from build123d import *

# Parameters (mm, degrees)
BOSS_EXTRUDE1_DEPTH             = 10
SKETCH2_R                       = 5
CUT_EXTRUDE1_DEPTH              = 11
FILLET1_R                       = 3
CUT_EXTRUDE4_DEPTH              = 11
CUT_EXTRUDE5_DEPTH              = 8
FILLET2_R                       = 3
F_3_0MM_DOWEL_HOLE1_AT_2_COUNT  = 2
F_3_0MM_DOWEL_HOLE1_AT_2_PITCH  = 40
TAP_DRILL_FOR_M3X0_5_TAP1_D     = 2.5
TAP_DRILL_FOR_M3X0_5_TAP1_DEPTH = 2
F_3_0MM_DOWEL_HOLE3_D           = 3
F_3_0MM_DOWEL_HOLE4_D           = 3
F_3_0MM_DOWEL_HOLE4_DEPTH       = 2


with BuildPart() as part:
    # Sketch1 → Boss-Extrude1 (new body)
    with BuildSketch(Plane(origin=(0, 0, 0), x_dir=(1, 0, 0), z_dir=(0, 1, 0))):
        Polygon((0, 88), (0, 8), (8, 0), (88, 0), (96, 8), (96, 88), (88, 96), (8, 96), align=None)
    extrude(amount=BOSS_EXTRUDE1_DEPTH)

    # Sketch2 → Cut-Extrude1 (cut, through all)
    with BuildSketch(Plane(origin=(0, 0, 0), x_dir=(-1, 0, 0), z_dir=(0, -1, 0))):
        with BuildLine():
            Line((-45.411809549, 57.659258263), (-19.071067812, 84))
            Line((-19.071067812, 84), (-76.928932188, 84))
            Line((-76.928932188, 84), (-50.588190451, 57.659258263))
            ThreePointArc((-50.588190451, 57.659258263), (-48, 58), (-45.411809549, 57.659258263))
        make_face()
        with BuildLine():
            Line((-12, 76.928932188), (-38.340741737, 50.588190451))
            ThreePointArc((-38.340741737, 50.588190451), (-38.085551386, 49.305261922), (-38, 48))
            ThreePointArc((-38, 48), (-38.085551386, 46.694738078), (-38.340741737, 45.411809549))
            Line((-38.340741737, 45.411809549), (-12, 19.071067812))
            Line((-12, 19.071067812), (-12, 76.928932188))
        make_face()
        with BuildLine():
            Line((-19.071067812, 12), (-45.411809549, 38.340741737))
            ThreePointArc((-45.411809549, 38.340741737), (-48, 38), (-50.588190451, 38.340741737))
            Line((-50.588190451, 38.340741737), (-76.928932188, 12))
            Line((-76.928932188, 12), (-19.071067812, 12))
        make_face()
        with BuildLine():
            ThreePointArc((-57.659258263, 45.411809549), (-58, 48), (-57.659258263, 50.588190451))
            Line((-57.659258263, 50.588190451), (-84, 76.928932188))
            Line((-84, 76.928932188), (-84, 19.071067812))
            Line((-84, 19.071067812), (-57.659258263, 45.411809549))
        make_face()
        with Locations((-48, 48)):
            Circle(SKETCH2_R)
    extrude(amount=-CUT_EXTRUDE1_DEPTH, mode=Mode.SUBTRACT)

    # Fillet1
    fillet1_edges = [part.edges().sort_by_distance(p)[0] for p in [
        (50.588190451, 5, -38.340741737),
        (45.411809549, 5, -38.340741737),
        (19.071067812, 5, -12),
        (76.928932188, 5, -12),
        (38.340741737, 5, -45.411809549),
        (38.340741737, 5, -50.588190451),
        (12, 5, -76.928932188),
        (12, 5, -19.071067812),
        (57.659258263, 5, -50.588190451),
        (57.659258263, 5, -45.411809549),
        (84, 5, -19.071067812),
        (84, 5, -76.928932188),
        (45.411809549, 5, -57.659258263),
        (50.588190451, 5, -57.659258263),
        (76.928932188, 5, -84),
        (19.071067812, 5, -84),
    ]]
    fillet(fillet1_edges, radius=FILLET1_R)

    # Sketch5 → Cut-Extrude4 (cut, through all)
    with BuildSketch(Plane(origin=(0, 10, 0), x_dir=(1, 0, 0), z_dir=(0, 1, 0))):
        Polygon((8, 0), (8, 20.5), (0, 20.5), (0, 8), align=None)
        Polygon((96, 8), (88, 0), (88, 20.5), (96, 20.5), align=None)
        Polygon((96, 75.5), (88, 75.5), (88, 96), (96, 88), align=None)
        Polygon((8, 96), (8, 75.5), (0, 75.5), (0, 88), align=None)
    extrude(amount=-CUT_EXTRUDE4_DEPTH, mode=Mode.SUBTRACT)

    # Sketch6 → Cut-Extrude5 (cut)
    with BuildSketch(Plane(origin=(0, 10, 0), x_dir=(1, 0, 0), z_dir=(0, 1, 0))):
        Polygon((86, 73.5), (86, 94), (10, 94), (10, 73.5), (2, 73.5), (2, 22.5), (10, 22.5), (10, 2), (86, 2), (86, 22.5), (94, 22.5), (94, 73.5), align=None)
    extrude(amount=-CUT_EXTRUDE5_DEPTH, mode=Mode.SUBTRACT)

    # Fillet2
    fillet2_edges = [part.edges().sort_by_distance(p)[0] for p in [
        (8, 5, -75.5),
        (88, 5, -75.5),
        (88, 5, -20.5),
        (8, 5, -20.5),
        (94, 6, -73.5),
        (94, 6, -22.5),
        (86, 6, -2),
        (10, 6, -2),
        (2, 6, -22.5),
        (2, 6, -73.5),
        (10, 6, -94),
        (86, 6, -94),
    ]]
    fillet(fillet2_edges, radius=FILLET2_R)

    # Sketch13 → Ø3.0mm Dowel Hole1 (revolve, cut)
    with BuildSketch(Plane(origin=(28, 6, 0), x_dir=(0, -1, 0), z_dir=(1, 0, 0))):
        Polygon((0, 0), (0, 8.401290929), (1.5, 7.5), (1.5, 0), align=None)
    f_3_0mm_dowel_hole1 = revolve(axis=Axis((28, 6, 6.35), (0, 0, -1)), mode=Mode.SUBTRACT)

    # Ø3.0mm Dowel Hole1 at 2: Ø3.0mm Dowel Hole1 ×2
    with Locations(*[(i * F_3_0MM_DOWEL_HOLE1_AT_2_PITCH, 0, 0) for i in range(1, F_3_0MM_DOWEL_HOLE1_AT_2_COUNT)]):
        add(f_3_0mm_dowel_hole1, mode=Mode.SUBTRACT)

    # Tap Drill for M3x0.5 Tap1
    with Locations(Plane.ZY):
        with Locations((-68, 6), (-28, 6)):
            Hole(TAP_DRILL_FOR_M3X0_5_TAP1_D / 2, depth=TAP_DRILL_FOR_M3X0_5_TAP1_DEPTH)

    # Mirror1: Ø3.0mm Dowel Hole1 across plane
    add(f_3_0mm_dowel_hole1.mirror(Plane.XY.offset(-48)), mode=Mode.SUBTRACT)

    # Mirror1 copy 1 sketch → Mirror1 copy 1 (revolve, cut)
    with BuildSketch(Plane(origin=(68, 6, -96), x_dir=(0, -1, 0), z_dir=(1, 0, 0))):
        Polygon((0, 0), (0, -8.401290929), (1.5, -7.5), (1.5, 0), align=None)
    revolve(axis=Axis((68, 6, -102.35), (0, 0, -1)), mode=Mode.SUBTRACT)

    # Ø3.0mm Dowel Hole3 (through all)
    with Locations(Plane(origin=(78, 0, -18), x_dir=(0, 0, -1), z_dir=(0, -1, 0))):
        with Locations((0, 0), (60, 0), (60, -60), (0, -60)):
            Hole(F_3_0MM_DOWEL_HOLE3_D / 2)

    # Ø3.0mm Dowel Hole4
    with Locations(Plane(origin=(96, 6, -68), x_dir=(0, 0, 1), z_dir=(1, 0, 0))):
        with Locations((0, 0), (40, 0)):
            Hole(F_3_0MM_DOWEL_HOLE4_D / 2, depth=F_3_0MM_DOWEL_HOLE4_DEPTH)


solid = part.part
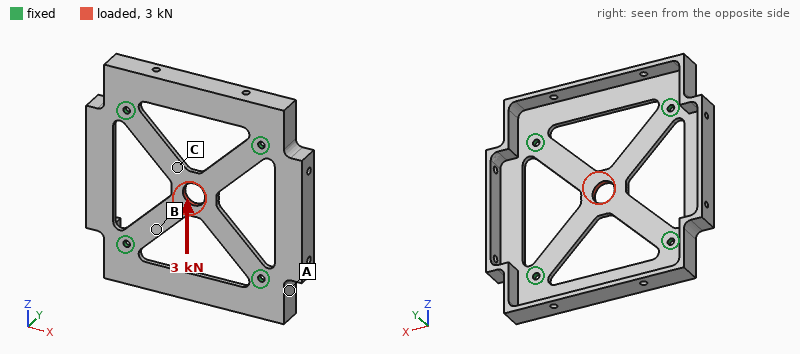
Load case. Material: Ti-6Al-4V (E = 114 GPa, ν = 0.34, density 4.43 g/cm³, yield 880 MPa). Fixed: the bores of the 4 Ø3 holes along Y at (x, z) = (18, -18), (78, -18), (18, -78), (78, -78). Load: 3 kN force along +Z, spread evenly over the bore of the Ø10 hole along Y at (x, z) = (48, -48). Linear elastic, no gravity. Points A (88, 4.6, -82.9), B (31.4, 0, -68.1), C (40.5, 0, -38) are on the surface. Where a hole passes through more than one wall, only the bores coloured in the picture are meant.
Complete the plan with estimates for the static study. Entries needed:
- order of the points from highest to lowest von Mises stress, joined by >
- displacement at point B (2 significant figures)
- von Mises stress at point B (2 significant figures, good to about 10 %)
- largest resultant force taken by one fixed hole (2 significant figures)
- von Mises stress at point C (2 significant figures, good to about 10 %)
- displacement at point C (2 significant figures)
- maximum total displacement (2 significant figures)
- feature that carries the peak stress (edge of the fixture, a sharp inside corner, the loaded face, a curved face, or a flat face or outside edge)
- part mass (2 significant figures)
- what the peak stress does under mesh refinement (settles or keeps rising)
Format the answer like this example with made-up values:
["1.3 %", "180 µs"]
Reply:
["B > C > A", "11 µm", "55 MPa", "980 N", "45 MPa", "21 µm", "27 µm", "edge of the fixture", "73 g", "keeps rising"]
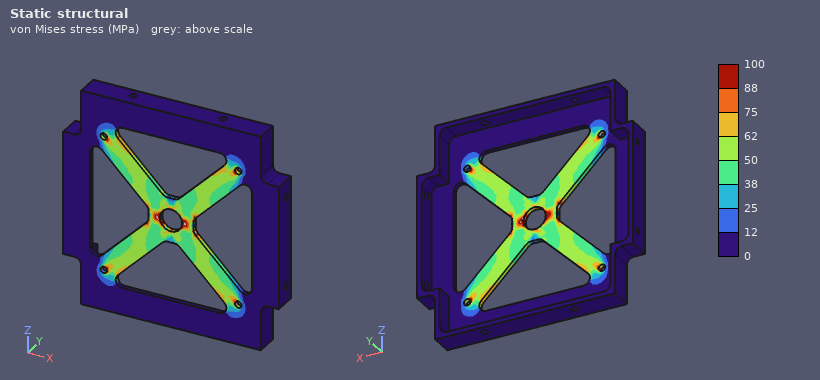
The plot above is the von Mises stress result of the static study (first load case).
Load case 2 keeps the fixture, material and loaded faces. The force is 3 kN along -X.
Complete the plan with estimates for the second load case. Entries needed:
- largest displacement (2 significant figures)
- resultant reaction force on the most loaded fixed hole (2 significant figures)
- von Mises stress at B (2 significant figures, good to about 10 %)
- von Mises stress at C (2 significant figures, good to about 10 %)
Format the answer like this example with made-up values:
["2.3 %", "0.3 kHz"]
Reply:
["27 µm", "980 N", "48 MPa", "50 MPa"]
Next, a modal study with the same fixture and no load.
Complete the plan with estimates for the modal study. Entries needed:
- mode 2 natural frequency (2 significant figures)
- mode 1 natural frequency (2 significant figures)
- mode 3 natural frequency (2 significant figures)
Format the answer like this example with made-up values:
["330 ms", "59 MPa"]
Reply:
["2300 Hz", "1800 Hz", "2500 Hz"]
